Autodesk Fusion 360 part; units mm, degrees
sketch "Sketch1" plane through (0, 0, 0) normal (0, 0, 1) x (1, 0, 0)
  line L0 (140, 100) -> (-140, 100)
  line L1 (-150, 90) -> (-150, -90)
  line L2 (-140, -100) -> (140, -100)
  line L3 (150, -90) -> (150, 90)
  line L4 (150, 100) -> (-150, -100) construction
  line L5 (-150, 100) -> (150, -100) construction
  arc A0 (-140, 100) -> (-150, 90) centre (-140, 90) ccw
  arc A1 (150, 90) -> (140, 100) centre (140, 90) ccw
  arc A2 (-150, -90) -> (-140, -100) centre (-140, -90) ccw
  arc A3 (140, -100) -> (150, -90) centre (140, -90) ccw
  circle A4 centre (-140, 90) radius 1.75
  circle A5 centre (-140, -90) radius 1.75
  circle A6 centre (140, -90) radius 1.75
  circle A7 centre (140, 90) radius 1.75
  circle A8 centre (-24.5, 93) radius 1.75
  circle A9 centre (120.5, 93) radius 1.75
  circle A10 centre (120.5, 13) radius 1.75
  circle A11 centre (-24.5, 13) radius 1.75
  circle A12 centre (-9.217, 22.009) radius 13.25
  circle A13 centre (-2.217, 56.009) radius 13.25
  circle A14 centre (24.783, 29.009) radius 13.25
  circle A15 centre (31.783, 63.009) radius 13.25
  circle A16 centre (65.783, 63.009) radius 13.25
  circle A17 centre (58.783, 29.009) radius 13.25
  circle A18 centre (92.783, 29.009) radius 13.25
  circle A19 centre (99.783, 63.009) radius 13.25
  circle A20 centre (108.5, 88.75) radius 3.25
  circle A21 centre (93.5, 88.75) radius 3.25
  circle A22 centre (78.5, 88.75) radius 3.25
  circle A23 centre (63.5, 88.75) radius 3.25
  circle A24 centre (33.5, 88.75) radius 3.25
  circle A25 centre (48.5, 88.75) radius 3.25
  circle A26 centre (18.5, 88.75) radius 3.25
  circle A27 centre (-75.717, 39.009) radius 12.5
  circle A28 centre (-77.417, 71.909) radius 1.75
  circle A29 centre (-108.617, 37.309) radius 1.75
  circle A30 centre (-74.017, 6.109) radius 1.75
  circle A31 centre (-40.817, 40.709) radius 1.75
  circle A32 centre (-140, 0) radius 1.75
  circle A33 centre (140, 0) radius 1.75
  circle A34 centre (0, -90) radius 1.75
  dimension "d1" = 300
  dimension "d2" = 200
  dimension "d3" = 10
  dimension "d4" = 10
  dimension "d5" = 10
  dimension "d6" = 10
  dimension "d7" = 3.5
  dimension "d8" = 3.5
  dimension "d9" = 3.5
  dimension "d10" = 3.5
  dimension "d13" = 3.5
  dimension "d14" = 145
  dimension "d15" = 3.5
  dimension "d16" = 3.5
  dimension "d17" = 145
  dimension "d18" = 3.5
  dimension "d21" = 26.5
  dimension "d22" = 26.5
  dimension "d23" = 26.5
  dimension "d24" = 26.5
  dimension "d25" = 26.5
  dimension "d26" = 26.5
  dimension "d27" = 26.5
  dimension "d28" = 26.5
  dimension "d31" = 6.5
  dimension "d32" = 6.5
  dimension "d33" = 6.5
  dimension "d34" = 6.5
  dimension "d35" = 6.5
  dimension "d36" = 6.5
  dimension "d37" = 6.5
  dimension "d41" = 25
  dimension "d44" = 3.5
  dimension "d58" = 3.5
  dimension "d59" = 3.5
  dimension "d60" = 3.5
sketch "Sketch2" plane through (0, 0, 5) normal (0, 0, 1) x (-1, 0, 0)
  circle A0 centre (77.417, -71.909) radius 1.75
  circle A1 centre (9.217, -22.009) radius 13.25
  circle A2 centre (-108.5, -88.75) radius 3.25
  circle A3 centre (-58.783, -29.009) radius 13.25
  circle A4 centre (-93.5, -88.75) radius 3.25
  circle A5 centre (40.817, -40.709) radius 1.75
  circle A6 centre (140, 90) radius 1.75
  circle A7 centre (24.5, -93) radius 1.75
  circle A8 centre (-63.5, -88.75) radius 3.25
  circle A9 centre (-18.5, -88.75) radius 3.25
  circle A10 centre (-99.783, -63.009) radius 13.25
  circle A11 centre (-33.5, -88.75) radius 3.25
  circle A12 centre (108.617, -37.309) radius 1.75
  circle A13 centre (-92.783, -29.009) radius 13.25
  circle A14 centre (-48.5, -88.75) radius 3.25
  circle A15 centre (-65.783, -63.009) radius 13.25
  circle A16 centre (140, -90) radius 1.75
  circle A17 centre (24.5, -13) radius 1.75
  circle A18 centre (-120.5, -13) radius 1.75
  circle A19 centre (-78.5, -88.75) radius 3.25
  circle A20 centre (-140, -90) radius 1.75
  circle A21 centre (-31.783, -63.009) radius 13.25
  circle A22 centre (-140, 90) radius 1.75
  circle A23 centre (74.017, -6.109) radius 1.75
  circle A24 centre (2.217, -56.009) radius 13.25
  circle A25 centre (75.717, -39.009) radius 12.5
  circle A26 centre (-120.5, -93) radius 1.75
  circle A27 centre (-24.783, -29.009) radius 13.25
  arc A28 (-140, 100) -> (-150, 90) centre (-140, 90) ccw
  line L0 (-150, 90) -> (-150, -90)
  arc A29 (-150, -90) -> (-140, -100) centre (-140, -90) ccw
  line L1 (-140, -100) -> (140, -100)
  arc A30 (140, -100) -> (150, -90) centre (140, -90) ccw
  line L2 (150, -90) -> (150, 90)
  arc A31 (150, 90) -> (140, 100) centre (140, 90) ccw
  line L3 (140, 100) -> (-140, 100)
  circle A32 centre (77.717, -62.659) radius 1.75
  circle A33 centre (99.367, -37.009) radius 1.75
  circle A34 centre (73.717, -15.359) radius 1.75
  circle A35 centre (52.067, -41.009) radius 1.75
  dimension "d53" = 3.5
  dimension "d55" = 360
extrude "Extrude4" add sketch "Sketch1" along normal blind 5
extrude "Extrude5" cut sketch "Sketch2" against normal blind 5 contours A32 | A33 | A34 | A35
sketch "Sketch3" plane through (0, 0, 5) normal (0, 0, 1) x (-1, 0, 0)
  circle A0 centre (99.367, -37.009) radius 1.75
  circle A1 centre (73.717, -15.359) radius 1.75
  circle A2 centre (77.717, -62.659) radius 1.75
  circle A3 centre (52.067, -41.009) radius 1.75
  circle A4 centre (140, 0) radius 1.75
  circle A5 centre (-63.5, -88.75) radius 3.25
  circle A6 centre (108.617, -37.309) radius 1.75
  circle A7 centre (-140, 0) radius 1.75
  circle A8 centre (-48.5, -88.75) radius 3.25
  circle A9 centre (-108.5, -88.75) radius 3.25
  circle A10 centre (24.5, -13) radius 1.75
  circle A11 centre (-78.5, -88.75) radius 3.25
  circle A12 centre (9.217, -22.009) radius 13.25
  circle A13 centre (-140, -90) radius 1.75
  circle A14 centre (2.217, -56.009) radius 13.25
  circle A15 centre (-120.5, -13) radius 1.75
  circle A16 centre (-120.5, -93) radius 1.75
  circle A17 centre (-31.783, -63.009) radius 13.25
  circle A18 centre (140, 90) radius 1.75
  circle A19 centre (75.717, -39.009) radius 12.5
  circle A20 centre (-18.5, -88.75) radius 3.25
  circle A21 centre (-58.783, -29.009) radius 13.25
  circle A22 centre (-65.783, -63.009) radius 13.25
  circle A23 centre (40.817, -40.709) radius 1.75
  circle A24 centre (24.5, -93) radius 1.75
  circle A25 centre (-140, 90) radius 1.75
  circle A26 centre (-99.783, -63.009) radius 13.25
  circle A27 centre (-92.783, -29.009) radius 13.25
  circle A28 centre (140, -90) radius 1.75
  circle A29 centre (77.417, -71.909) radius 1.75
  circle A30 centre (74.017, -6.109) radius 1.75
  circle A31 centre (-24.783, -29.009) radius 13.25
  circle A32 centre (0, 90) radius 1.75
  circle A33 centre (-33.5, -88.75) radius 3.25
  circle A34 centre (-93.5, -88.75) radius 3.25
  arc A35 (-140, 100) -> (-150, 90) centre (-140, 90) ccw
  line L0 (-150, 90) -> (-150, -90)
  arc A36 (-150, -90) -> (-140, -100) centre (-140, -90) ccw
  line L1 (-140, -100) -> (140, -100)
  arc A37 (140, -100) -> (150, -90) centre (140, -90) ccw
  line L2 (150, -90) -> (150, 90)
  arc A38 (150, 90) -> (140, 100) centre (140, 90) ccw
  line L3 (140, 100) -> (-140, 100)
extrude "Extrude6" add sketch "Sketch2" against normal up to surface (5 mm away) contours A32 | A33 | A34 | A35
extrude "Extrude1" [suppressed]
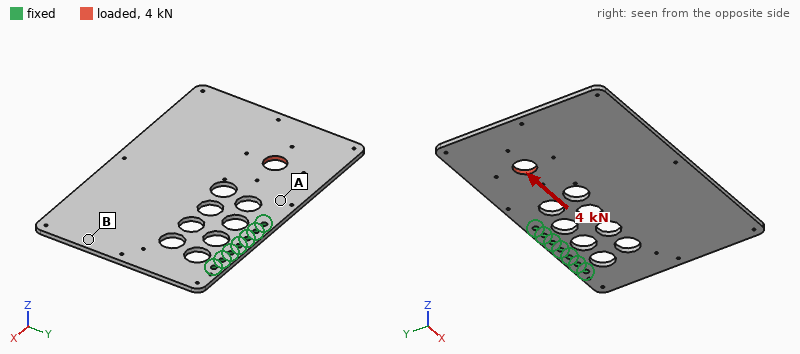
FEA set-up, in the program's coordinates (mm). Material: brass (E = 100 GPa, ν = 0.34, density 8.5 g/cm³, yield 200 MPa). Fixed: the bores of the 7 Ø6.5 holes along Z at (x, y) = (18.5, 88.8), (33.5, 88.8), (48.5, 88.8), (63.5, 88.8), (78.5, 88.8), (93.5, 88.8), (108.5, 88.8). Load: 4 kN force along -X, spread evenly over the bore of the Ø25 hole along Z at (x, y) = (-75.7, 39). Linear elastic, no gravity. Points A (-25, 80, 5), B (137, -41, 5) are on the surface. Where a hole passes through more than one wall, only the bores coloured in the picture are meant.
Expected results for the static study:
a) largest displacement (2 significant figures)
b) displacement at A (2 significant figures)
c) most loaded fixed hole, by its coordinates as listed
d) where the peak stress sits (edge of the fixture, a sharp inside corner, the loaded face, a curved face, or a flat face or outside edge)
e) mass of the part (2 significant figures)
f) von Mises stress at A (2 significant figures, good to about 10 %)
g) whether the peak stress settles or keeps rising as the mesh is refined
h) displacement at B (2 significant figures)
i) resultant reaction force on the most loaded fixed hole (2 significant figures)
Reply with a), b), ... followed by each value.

a) 0.12 mm
b) 0.030 mm
c) (18.5, 88.8)
d) edge of the fixture
e) 2.3 kg
f) 14 MPa
g) keeps rising
h) 0.068 mm
i) 2.8 kN
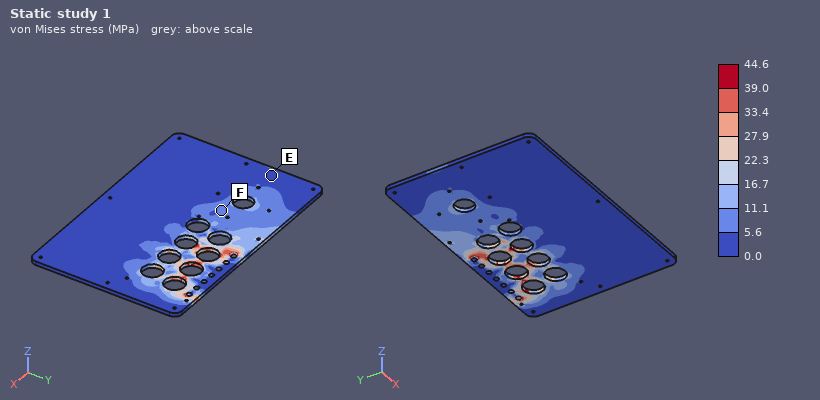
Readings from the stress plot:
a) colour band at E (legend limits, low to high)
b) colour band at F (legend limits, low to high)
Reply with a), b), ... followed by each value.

a) 0.0 to 5.6 MPa
b) 5.6 to 11.1 MPa
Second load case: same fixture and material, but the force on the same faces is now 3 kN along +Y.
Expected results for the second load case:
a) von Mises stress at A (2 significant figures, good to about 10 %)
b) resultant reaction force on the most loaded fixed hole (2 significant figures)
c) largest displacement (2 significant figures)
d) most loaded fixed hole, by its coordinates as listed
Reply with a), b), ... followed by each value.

a) 8.4 MPa
b) 5.7 kN
c) 0.22 mm
d) (18.5, 88.8)
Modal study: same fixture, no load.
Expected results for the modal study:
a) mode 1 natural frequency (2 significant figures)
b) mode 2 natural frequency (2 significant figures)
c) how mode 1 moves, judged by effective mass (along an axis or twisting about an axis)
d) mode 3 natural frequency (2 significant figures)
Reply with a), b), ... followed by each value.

a) 41 Hz
b) 74 Hz
c) along Z
d) 170 Hz
